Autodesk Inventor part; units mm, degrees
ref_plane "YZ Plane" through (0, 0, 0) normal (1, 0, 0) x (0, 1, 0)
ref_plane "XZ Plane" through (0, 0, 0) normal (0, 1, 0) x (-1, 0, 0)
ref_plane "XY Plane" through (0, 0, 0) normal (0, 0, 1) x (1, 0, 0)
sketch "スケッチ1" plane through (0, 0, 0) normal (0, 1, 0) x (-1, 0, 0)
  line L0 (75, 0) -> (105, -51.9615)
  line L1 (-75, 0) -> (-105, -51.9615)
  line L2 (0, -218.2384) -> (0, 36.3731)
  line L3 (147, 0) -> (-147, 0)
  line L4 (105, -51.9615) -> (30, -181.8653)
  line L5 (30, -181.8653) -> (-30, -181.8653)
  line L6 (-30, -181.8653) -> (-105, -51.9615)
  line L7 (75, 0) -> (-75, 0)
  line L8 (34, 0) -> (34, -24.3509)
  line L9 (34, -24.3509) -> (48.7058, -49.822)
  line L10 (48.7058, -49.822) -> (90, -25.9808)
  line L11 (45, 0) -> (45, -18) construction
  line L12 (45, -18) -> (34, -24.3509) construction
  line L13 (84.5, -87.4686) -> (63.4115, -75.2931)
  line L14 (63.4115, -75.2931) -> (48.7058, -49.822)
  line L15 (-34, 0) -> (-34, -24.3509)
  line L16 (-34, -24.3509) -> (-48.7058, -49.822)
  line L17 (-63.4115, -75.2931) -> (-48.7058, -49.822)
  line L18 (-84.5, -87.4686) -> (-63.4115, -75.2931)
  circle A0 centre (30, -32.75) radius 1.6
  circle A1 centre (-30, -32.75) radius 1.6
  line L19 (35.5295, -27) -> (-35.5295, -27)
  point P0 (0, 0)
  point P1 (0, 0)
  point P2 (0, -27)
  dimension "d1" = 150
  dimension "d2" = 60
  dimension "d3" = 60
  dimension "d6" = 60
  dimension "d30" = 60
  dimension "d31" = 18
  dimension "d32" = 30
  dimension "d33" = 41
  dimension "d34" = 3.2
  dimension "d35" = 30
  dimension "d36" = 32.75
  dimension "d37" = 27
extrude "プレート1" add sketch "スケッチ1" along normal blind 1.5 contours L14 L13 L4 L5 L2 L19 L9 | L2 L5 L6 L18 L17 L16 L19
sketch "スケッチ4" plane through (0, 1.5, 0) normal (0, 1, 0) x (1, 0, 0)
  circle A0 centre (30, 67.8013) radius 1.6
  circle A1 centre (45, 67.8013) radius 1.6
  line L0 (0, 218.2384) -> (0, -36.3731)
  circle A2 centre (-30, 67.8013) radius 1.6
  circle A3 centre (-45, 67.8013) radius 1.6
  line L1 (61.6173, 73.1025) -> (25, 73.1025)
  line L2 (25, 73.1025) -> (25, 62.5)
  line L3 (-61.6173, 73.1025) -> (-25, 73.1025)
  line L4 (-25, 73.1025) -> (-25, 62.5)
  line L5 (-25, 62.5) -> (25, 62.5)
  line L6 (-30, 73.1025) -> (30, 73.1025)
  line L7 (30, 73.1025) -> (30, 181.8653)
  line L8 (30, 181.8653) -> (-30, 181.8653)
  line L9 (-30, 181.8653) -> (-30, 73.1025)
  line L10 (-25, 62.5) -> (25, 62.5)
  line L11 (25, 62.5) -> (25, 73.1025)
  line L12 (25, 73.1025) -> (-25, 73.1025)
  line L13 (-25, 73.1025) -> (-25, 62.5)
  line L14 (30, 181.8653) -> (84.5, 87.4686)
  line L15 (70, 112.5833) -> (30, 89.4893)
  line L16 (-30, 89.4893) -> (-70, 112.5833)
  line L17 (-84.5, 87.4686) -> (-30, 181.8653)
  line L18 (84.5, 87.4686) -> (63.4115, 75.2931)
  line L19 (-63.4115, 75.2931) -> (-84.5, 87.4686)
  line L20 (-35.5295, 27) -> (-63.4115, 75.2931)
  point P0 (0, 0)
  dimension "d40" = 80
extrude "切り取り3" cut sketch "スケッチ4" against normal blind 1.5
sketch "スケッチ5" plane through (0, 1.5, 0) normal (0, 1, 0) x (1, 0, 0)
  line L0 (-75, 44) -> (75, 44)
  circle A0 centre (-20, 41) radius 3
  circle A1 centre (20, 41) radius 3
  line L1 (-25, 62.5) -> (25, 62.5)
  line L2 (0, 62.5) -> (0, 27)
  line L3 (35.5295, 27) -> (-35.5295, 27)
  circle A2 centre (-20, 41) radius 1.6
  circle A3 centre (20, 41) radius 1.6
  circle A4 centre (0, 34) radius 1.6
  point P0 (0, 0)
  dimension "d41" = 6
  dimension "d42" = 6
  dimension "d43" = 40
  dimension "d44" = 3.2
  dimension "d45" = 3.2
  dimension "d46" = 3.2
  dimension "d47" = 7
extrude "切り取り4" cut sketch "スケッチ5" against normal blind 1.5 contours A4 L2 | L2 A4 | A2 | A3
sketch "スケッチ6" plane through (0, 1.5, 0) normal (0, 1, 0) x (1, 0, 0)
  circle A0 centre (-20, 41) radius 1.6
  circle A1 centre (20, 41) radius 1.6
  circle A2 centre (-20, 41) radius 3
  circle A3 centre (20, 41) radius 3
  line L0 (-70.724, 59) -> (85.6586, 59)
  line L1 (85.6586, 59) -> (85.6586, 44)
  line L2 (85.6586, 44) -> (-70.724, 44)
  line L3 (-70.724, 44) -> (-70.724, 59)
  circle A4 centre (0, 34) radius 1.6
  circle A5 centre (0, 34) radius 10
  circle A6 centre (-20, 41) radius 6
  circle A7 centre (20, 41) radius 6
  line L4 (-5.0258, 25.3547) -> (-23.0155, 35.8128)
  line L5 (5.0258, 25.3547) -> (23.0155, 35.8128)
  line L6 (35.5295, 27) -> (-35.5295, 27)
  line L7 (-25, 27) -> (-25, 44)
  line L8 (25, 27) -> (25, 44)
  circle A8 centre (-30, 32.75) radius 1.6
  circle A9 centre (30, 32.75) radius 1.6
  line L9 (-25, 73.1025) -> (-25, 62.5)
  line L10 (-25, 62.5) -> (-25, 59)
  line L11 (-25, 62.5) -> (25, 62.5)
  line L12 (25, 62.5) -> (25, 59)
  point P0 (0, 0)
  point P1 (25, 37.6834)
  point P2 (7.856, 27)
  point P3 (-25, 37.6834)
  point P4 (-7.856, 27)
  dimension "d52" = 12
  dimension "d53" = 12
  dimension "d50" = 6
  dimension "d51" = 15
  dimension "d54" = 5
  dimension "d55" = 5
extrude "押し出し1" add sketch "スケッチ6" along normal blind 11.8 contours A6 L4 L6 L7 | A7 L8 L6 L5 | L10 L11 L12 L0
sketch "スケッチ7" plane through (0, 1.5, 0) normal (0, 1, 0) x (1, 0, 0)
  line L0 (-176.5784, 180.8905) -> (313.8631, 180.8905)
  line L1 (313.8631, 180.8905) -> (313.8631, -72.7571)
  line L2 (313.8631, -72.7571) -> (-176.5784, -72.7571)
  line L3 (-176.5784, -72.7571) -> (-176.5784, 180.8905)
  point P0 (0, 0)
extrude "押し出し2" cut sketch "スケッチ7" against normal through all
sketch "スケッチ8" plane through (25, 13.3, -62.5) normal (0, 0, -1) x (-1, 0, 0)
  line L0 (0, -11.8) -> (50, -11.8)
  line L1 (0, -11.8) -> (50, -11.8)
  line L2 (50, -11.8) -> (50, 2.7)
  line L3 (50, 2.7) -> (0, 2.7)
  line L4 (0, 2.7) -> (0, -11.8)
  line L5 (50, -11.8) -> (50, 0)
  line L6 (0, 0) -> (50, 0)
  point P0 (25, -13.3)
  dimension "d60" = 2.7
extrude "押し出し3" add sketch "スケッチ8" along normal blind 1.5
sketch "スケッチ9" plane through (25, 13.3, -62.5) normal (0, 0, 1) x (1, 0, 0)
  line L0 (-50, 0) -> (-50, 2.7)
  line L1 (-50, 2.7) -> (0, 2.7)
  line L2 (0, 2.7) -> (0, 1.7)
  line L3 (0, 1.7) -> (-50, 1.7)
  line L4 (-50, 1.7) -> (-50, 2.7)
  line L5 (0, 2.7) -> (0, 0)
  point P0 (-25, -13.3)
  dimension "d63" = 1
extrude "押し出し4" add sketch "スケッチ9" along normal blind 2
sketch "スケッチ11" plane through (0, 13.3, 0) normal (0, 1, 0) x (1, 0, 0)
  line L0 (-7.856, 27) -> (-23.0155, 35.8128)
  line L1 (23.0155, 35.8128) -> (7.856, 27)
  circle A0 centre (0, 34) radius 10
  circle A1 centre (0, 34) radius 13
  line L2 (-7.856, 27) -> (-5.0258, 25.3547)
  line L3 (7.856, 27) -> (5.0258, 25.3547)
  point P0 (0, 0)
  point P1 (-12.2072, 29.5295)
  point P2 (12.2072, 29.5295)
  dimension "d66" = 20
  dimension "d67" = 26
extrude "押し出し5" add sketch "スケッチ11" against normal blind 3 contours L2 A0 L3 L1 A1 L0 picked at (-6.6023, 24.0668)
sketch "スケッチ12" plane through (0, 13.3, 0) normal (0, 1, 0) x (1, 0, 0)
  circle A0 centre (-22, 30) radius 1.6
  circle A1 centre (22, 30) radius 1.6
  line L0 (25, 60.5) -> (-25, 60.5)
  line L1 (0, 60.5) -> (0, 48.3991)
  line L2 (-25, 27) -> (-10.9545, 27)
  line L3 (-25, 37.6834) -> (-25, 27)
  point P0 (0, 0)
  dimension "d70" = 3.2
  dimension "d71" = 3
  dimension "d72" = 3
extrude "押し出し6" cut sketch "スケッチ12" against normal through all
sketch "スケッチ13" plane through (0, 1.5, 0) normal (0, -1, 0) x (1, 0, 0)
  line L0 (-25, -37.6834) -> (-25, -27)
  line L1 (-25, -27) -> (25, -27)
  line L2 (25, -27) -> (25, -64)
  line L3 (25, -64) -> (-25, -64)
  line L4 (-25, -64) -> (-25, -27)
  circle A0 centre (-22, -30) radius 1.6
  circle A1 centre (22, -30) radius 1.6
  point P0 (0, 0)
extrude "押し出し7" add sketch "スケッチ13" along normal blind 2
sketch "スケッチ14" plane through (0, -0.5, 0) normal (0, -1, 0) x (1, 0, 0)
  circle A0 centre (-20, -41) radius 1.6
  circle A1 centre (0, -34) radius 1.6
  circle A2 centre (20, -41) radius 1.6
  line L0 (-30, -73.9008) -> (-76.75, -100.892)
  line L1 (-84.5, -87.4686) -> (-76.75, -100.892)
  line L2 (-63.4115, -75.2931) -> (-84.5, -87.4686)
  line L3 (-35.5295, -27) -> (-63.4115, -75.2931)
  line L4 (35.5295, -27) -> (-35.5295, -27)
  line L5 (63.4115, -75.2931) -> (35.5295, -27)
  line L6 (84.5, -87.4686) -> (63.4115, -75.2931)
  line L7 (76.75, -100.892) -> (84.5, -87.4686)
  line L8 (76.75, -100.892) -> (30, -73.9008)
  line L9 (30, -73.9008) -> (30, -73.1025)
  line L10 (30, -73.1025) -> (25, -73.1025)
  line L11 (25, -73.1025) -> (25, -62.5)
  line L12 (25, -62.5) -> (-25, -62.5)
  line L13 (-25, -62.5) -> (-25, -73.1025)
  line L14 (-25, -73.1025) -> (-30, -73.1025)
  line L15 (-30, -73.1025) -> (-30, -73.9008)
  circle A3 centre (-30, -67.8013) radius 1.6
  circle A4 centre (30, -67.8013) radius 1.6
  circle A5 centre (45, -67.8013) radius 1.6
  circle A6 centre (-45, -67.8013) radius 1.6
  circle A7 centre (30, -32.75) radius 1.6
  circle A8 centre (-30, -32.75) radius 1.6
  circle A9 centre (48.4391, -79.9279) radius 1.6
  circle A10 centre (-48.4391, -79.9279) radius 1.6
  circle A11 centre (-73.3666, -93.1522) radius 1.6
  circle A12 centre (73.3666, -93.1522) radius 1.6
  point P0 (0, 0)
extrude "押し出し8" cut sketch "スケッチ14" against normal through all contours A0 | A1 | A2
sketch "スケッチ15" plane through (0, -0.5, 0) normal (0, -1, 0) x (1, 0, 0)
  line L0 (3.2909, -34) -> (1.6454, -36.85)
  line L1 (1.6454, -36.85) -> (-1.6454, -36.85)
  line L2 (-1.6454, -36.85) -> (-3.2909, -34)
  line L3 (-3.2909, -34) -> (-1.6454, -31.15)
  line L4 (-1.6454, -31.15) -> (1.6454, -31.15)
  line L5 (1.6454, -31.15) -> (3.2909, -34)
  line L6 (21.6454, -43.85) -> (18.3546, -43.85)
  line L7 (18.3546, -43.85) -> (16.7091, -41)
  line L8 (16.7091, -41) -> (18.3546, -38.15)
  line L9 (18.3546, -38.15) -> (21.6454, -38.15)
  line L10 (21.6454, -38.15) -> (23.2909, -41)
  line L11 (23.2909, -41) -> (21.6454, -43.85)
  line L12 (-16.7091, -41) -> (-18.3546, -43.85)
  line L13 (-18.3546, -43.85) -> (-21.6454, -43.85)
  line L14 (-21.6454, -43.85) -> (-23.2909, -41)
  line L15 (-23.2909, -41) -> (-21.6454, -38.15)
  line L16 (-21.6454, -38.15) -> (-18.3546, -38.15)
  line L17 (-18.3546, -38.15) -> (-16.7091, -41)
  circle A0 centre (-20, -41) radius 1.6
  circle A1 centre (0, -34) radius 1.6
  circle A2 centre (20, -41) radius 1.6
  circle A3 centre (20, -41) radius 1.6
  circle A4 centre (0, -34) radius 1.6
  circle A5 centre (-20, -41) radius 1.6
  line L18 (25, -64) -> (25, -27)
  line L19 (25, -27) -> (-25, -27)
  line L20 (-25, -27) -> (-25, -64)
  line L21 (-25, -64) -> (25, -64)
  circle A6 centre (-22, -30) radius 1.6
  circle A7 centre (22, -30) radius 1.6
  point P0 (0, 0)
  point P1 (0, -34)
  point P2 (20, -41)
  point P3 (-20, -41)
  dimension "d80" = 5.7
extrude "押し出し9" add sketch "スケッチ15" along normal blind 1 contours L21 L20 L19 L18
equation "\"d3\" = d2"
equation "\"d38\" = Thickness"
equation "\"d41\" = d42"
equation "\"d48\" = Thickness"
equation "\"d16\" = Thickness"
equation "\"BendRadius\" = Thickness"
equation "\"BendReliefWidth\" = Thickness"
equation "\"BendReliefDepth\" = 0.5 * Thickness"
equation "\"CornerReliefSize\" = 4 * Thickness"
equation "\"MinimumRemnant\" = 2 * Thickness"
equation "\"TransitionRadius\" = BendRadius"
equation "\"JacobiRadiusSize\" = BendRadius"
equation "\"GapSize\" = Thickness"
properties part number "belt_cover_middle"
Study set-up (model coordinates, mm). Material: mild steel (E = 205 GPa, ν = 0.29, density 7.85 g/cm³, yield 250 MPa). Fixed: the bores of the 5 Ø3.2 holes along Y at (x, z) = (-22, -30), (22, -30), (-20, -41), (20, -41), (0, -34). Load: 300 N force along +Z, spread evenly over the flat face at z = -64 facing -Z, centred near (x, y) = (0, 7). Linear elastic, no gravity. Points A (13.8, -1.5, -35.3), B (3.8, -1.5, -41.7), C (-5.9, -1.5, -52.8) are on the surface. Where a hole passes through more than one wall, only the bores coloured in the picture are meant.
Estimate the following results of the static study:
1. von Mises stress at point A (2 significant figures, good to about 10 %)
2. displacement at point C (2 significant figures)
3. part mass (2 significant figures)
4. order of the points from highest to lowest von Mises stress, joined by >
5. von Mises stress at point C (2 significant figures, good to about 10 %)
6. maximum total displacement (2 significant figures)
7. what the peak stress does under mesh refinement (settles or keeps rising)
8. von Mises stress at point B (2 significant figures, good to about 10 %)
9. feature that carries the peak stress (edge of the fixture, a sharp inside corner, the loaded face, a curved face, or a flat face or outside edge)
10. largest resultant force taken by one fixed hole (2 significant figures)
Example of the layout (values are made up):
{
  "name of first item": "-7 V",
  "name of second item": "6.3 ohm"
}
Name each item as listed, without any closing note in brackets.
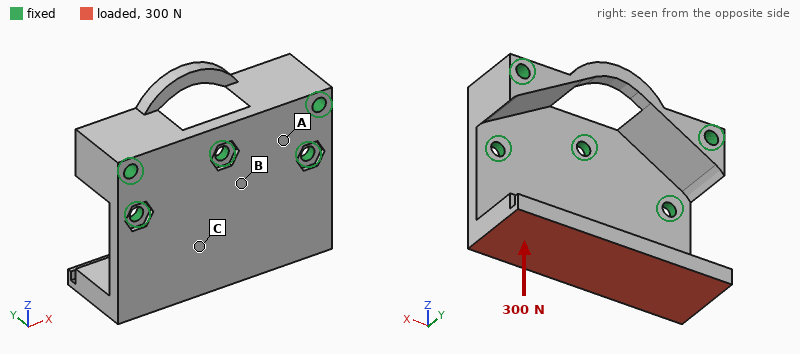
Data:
{
  "von Mises stress at point A": "7.1 MPa",
  "displacement at point C": "10 µm",
  "part mass": "84 g",
  "order of the points from highest to lowest von Mises stress, joined by >": "C > B > A",
  "von Mises stress at point C": "25 MPa",
  "maximum total displacement": "44 µm",
  "what the peak stress does under mesh refinement": "keeps rising",
  "von Mises stress at point B": "17 MPa",
  "feature that carries the peak stress": "edge of the fixture",
  "largest resultant force taken by one fixed hole": "150 N"
}
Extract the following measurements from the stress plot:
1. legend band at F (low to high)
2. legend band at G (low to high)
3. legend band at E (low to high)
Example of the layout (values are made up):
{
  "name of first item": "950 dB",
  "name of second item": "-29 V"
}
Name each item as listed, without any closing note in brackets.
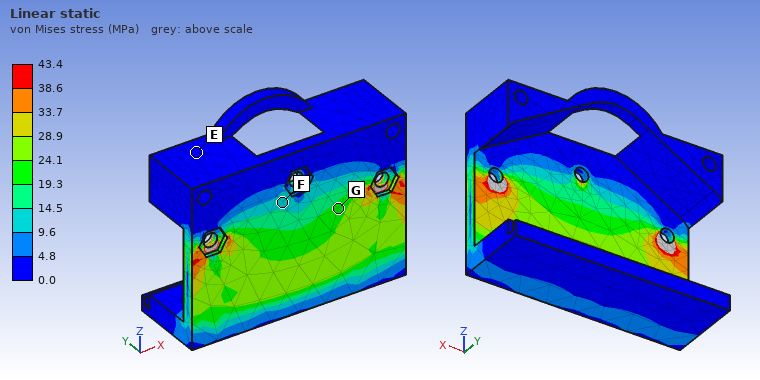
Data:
{
  "legend band at F": "9.6 to 14.5 MPa",
  "legend band at G": "19.3 to 24.1 MPa",
  "legend band at E": "0.0 to 4.8 MPa"
}
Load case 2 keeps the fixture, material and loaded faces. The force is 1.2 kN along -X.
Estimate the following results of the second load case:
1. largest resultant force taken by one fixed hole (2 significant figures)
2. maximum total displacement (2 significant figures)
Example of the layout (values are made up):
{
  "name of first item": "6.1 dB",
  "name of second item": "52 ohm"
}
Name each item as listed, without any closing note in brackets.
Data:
{
  "largest resultant force taken by one fixed hole": "700 N",
  "maximum total displacement": "45 µm"
}
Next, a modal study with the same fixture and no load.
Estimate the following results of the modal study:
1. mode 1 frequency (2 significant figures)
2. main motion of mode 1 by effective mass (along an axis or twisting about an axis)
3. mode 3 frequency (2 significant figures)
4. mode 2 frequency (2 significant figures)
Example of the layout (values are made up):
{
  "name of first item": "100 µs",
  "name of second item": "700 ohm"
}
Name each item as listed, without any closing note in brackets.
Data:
{
  "mode 1 frequency": "1800 Hz",
  "main motion of mode 1 by effective mass": "along Y",
  "mode 3 frequency": "7200 Hz",
  "mode 2 frequency": "3900 Hz"
}
